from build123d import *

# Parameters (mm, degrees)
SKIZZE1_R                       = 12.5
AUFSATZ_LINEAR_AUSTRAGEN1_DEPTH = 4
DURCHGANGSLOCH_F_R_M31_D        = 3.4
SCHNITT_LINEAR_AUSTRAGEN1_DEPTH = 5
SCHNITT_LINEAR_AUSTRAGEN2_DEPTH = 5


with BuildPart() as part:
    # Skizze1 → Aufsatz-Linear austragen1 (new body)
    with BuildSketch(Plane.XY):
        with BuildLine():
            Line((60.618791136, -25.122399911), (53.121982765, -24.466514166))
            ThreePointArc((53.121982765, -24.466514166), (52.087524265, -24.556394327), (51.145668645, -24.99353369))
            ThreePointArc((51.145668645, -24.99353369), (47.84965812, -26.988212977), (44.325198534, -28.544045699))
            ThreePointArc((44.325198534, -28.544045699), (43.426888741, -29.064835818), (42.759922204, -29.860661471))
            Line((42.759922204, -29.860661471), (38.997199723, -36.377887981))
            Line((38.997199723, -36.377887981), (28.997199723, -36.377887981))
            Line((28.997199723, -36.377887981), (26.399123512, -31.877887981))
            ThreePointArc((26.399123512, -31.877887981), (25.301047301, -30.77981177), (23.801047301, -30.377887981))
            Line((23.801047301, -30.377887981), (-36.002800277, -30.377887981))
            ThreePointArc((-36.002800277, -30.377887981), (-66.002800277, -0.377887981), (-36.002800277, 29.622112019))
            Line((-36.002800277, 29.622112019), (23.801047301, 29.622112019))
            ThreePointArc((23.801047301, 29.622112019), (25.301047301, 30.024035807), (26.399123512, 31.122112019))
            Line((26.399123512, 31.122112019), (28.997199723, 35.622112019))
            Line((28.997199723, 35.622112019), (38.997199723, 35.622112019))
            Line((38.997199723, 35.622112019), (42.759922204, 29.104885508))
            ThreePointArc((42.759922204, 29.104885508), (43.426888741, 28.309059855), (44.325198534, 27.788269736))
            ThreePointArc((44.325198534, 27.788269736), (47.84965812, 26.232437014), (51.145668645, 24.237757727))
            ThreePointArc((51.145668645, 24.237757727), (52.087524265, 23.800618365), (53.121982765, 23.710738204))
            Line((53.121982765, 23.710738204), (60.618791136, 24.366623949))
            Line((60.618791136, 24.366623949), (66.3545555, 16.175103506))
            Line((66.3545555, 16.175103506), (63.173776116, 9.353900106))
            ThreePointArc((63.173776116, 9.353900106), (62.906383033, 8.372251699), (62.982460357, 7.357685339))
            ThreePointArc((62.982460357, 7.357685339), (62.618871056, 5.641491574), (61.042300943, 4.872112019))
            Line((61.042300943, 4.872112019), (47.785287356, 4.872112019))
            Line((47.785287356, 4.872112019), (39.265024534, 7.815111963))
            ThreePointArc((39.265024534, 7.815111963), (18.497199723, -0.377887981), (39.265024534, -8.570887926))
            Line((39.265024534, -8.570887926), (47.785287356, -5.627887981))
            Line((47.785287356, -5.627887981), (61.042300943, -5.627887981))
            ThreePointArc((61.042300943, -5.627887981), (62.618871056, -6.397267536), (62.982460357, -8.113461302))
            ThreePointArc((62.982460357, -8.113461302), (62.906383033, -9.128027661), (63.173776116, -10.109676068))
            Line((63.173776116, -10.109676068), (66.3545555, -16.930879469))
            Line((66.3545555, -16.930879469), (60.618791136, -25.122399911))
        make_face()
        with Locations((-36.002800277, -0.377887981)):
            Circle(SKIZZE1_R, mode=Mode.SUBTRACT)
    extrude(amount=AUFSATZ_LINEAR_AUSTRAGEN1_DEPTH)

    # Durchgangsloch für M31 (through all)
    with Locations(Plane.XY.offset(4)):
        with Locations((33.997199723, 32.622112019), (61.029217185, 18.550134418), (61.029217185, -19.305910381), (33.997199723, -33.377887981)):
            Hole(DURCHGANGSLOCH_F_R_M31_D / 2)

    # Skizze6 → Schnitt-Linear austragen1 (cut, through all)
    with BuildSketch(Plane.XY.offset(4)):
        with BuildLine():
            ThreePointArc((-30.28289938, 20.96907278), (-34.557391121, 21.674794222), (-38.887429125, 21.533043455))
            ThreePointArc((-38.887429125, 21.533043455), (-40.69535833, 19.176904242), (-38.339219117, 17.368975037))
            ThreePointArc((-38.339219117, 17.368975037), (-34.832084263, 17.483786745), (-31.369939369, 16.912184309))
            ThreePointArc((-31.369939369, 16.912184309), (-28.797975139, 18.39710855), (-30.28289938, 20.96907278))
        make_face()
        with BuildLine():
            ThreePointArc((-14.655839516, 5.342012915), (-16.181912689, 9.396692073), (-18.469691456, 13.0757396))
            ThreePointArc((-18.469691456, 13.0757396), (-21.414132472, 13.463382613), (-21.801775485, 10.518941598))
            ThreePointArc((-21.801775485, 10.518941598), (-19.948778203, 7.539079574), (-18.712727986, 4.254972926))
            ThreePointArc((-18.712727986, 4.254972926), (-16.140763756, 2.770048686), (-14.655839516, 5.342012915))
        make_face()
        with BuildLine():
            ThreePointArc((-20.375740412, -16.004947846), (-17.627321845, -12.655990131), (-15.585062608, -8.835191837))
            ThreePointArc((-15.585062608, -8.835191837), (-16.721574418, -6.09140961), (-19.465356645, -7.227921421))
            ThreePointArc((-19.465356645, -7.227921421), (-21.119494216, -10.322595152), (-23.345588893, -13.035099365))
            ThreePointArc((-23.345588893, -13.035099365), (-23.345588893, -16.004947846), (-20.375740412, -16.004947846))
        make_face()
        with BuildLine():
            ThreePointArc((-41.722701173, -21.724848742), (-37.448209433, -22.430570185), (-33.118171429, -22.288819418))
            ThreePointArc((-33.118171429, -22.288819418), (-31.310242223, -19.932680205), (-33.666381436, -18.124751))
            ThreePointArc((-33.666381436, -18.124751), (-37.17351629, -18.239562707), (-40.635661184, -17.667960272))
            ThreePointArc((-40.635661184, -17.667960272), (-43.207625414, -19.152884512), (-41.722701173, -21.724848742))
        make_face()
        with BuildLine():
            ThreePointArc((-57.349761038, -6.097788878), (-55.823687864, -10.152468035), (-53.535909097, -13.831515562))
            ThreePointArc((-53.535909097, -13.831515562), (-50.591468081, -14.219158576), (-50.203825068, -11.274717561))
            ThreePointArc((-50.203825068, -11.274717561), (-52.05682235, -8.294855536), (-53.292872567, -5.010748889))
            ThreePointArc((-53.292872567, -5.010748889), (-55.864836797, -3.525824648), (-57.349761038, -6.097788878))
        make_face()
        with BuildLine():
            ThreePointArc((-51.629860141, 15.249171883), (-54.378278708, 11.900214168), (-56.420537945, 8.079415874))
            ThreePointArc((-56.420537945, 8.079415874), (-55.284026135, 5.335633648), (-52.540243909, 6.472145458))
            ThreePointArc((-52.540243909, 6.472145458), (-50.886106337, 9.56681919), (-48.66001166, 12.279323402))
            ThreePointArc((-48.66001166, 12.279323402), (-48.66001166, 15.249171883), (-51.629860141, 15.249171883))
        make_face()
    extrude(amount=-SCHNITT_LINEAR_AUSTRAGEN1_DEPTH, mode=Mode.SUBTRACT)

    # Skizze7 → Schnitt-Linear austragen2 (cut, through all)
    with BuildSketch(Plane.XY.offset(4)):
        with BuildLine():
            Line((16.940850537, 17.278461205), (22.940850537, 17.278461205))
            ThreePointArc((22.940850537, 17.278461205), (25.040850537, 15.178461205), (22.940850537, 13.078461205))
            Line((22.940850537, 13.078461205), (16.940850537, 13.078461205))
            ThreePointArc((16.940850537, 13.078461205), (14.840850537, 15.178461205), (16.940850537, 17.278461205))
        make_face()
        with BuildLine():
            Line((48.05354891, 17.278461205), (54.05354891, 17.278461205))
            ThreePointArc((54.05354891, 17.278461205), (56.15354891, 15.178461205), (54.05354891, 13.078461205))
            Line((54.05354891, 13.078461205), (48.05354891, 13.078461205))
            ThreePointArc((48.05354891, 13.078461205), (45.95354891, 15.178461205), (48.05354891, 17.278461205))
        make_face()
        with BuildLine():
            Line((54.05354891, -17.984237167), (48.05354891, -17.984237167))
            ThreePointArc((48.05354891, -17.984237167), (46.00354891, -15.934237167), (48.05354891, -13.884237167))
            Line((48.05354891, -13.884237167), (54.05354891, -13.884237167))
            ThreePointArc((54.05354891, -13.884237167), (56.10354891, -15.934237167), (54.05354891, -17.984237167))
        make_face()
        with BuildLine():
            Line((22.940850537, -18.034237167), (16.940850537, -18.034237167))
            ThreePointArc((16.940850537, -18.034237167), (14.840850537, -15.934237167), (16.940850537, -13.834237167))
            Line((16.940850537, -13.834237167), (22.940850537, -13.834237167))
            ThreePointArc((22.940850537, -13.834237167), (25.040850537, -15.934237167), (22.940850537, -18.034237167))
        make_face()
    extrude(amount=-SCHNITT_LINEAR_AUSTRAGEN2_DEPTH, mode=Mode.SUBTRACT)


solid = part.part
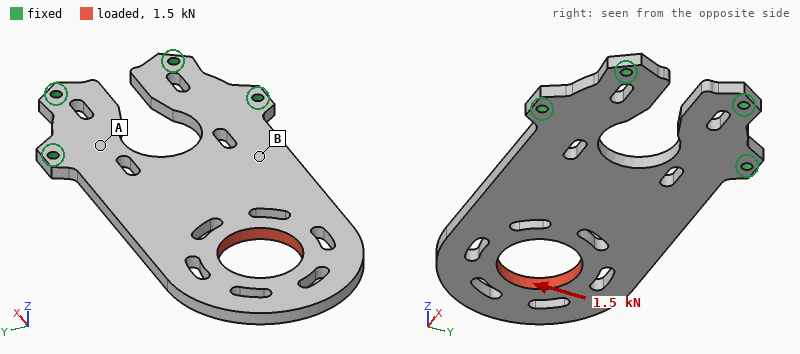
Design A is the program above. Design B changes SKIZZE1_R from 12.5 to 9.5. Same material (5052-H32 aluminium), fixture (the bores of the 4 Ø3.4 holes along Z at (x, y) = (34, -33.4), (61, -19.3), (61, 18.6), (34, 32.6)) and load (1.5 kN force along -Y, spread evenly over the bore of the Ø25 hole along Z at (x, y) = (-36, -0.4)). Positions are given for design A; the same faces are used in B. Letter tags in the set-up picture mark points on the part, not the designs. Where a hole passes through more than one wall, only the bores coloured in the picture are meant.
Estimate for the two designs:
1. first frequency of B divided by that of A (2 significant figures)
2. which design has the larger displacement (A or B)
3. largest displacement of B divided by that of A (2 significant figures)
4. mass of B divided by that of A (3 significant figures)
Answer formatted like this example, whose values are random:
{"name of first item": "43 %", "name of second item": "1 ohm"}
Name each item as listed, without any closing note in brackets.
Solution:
{"first frequency of B divided by that of A": "0.96", "which design has the larger displacement": "A", "largest displacement of B divided by that of A": "0.90", "mass of B divided by that of A": "1.04"}
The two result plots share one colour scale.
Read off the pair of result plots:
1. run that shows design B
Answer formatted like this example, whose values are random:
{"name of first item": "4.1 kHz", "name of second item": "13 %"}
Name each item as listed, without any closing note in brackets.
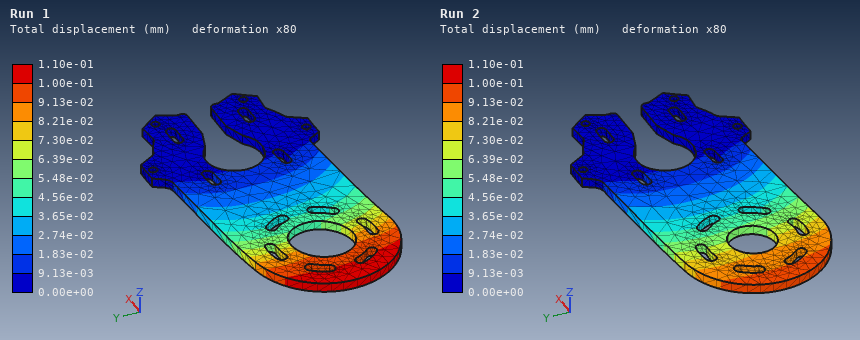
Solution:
{"run that shows design B": "Run 2"}
